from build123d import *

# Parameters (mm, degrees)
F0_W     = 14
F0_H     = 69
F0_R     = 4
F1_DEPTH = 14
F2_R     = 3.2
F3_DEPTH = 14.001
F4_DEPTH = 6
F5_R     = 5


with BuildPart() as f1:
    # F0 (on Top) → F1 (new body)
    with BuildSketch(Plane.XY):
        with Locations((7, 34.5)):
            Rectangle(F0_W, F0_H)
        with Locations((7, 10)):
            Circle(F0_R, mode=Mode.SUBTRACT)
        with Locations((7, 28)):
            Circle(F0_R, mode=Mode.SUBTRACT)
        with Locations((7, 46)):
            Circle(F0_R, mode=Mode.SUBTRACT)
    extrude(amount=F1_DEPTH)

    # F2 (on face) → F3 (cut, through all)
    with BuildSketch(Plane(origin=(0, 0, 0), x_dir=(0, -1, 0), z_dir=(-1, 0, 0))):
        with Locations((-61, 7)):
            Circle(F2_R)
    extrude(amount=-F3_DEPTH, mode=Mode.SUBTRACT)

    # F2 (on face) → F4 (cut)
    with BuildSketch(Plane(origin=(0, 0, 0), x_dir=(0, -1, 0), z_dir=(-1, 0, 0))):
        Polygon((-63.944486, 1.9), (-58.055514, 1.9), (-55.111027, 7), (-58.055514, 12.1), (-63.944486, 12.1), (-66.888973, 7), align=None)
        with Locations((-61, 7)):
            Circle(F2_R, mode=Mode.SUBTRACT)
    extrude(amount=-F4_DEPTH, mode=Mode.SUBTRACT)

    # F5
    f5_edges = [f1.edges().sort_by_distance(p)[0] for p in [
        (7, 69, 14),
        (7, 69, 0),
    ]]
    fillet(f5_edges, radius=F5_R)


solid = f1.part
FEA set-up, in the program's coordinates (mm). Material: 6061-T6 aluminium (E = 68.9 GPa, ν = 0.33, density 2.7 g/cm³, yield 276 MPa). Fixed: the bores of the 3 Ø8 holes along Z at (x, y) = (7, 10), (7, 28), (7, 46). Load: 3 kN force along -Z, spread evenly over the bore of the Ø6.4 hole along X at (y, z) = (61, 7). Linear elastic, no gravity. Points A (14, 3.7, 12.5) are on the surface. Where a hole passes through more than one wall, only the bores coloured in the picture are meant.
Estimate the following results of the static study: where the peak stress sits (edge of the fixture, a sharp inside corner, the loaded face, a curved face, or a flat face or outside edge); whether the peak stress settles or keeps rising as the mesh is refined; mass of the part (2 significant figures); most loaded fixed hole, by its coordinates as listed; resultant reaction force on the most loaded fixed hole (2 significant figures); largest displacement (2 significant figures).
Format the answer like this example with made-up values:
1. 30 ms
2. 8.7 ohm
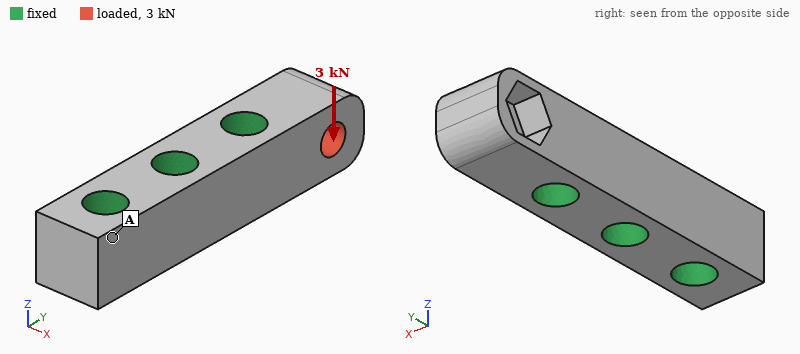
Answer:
1. edge of the fixture
2. keeps rising
3. 28 g
4. (7, 46)
5. 3.1 kN
6. 43 µm
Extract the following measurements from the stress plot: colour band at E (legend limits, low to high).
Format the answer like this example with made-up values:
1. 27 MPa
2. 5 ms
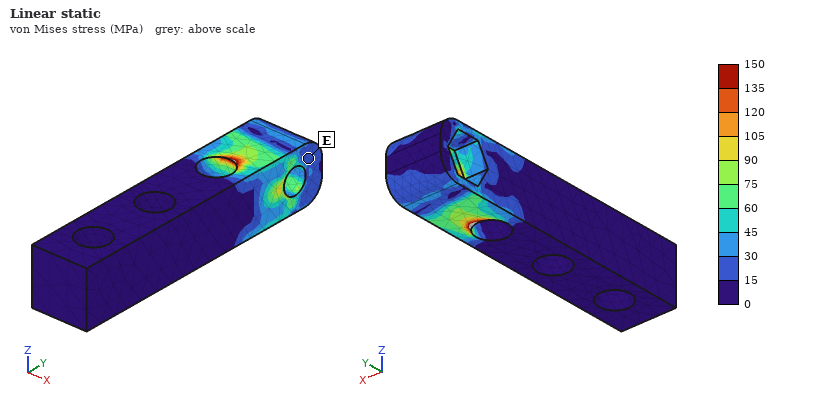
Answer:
1. 15 to 30 MPa
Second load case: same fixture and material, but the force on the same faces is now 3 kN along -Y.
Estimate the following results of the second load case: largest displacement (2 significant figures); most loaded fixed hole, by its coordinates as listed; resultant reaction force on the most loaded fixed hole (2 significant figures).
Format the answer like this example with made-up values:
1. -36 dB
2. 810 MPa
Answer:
1. 14 µm
2. (7, 46)
3. 2.9 kN
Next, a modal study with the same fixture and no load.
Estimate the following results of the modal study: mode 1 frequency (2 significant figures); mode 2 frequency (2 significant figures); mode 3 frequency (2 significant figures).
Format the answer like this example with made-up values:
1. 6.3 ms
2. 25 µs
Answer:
1. 19 kHz
2. 20 kHz
3. 33 kHz
